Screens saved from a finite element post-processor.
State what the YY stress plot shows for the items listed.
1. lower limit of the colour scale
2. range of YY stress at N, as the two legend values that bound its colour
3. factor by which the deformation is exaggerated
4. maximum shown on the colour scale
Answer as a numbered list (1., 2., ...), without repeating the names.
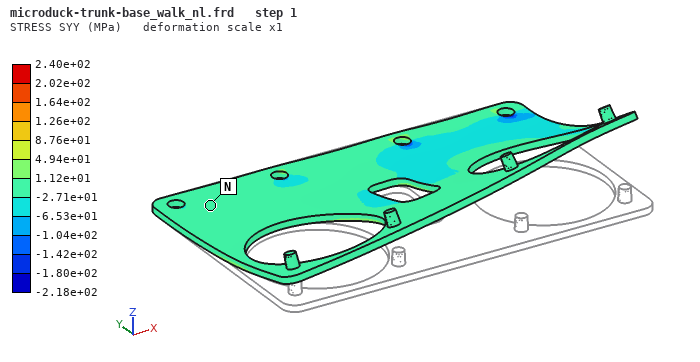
1. -2.18e+02 MPa
2. -2.71e+01 to 1.12e+01 MPa
3. 1
4. 2.40e+02 MPa
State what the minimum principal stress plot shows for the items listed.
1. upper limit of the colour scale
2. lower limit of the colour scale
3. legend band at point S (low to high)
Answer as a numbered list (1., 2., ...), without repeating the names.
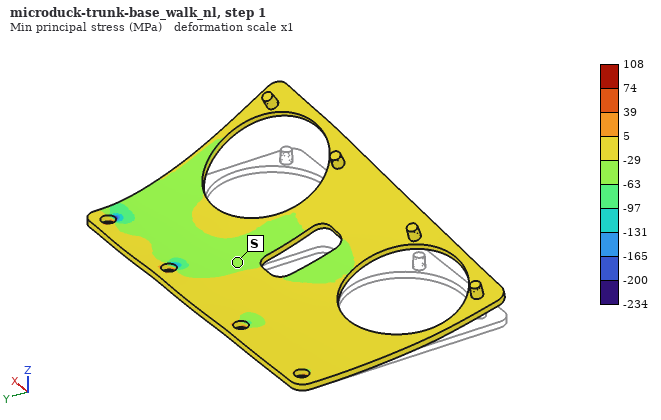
1. 108 MPa
2. -234 MPa
3. -63 to -29 MPa
